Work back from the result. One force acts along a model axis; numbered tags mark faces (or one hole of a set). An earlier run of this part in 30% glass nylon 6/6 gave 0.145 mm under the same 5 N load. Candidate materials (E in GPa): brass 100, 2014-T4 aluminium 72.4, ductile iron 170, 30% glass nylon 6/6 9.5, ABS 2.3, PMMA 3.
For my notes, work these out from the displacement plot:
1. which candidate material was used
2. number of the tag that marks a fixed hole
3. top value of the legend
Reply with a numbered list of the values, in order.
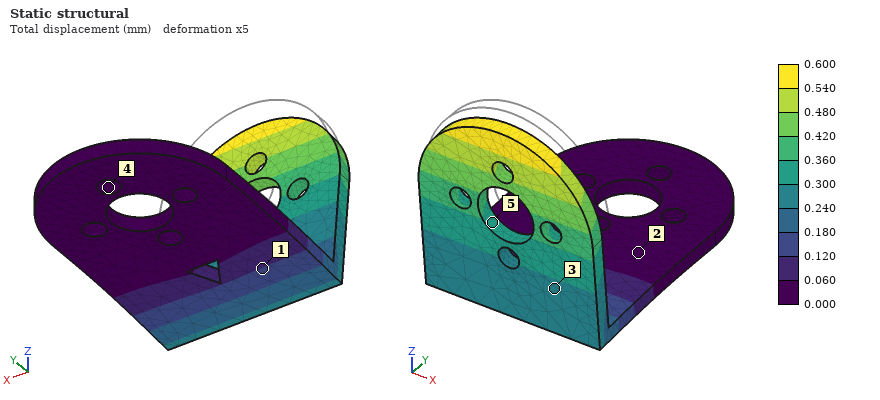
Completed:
1. ABS
2. 4
3. 0.600 mm
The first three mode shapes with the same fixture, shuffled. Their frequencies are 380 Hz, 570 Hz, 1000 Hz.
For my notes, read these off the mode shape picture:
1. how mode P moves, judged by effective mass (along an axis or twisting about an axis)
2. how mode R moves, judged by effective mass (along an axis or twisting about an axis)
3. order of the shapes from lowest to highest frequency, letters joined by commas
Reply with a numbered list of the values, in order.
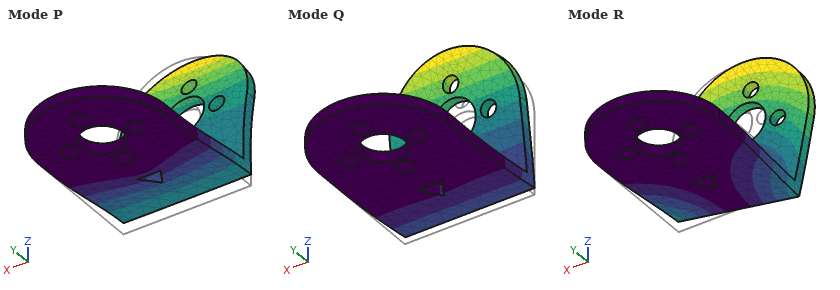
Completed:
1. along Z
2. along X
3. Q, R, P
